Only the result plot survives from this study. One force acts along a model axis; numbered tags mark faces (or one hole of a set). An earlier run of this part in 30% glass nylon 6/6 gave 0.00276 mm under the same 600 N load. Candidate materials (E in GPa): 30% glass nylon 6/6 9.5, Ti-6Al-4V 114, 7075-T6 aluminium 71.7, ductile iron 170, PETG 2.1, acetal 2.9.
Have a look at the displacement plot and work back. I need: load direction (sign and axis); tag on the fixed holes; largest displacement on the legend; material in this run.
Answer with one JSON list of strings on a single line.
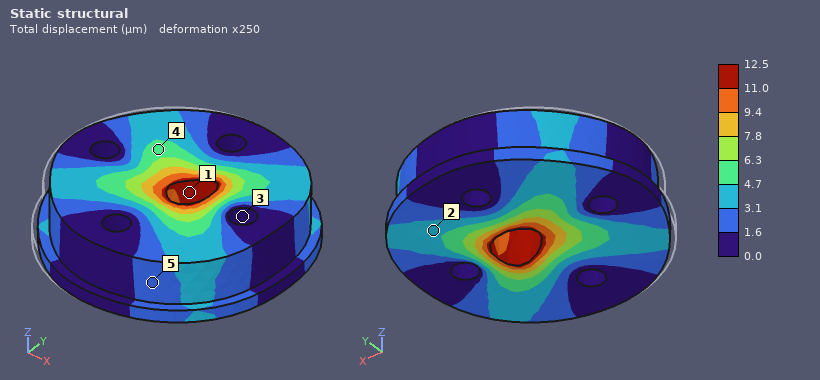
["+X", "3", "12.5 µm", "PETG"]
